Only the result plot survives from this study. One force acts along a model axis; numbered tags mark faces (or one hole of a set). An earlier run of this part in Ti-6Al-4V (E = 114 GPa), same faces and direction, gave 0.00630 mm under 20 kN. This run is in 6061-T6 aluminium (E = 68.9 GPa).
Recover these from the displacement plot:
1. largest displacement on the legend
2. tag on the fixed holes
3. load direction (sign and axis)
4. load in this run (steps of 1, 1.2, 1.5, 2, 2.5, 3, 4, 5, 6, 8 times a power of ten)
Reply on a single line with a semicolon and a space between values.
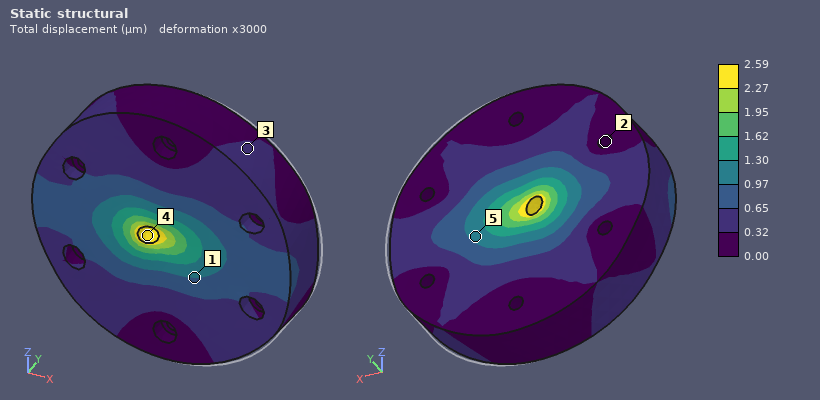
2.59 µm; 2; -X; 5 kN
